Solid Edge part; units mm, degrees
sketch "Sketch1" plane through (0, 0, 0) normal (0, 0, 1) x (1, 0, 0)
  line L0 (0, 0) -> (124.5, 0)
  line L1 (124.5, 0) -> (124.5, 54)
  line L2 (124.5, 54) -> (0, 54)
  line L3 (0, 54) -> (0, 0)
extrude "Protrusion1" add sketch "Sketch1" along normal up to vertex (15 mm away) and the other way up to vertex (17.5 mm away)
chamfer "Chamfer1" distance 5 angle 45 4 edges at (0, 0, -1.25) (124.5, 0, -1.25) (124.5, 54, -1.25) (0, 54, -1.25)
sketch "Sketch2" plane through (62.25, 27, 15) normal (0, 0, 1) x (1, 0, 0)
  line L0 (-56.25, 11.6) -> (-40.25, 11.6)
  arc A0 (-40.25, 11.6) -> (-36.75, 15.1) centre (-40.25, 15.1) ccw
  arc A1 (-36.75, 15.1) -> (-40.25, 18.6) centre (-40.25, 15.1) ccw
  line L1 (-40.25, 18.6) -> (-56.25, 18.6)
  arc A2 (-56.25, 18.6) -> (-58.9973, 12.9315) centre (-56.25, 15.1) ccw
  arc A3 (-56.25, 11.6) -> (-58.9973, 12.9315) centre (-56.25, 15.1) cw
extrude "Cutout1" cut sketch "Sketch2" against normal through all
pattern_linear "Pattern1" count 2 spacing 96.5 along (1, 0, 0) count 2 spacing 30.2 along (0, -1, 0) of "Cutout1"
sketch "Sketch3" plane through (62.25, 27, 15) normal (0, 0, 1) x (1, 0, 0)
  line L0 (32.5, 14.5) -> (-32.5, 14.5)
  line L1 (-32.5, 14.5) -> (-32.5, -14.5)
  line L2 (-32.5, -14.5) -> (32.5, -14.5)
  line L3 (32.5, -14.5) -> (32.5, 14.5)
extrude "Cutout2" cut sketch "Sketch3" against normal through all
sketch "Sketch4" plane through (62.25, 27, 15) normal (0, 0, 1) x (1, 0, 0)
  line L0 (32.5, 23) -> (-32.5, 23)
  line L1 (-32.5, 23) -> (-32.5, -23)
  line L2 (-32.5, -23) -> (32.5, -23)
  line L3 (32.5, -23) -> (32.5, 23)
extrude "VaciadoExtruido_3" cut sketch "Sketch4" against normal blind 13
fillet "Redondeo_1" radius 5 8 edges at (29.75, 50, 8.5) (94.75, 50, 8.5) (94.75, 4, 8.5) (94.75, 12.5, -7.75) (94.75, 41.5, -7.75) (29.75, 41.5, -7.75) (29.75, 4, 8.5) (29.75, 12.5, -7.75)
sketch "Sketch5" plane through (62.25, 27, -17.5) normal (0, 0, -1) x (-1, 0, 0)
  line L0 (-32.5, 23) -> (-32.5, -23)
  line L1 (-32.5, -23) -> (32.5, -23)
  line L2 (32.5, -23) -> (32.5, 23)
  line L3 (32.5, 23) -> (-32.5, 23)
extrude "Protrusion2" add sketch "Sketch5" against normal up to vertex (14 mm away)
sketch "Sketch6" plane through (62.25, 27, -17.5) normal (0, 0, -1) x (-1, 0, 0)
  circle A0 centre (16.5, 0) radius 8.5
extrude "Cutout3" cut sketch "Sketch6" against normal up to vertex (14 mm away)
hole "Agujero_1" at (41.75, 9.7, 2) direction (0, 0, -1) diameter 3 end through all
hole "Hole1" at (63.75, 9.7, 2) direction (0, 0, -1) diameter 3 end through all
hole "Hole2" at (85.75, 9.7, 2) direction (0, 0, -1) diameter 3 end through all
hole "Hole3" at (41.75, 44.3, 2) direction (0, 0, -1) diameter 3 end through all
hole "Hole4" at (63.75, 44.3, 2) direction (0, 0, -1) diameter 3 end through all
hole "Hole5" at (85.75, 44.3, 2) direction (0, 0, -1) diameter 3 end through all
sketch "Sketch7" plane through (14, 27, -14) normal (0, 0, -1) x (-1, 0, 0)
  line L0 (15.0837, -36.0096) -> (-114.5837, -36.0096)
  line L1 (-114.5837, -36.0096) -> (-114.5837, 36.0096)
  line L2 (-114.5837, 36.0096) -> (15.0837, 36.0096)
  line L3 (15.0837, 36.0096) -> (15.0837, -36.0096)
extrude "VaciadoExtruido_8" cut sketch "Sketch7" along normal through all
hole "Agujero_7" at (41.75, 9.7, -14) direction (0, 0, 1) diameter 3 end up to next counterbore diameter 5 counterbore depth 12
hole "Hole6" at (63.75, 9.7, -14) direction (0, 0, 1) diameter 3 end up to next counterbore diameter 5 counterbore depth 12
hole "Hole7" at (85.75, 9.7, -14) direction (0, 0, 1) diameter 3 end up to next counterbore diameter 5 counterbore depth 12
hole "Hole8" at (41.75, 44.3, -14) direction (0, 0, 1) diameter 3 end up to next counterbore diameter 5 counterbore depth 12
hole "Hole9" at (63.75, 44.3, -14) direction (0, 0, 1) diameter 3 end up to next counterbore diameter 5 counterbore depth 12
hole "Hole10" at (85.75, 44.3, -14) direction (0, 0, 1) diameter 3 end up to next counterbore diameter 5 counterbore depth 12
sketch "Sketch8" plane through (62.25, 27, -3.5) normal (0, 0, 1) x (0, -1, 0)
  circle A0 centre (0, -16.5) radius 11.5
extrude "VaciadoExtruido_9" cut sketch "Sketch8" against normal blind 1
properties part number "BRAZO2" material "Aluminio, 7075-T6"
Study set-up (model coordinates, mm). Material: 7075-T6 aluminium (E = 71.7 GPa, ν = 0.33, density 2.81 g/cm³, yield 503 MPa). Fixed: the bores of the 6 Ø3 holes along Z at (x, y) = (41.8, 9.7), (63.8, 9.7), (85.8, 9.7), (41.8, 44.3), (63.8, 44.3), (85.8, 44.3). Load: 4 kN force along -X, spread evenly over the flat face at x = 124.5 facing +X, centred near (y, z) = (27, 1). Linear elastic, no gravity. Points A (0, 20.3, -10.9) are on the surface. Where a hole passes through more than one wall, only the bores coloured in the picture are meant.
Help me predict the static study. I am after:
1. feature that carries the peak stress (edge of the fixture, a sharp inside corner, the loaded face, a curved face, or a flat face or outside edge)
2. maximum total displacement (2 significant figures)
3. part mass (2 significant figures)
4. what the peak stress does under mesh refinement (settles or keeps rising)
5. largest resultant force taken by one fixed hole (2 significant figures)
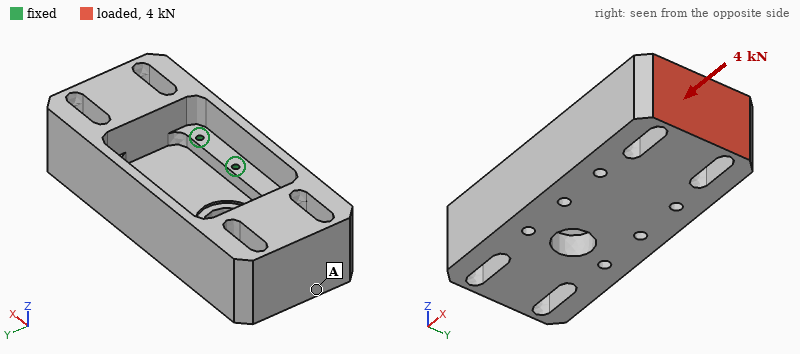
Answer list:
edge of the fixture
15 µm
350 g
keeps rising
1.2 kN
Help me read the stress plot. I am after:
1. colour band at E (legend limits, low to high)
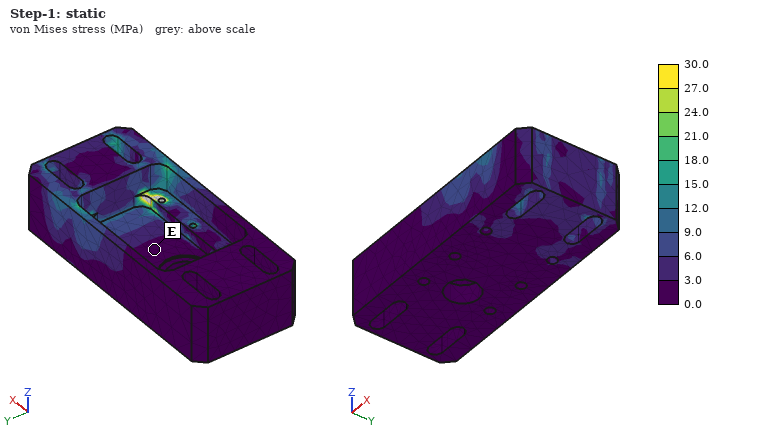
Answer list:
0.0 to 3.0 MPa
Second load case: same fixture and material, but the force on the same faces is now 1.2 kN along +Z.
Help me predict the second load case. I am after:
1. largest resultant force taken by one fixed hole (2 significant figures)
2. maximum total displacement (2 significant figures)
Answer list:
1.3 kN
34 µm
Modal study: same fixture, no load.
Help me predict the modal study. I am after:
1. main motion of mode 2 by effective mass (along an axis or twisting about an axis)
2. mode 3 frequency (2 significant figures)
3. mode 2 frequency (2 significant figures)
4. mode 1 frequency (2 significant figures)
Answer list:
along Z
6200 Hz
4600 Hz
3800 Hz
